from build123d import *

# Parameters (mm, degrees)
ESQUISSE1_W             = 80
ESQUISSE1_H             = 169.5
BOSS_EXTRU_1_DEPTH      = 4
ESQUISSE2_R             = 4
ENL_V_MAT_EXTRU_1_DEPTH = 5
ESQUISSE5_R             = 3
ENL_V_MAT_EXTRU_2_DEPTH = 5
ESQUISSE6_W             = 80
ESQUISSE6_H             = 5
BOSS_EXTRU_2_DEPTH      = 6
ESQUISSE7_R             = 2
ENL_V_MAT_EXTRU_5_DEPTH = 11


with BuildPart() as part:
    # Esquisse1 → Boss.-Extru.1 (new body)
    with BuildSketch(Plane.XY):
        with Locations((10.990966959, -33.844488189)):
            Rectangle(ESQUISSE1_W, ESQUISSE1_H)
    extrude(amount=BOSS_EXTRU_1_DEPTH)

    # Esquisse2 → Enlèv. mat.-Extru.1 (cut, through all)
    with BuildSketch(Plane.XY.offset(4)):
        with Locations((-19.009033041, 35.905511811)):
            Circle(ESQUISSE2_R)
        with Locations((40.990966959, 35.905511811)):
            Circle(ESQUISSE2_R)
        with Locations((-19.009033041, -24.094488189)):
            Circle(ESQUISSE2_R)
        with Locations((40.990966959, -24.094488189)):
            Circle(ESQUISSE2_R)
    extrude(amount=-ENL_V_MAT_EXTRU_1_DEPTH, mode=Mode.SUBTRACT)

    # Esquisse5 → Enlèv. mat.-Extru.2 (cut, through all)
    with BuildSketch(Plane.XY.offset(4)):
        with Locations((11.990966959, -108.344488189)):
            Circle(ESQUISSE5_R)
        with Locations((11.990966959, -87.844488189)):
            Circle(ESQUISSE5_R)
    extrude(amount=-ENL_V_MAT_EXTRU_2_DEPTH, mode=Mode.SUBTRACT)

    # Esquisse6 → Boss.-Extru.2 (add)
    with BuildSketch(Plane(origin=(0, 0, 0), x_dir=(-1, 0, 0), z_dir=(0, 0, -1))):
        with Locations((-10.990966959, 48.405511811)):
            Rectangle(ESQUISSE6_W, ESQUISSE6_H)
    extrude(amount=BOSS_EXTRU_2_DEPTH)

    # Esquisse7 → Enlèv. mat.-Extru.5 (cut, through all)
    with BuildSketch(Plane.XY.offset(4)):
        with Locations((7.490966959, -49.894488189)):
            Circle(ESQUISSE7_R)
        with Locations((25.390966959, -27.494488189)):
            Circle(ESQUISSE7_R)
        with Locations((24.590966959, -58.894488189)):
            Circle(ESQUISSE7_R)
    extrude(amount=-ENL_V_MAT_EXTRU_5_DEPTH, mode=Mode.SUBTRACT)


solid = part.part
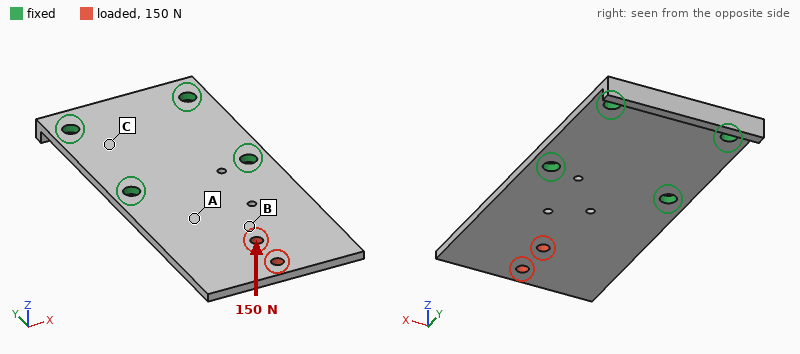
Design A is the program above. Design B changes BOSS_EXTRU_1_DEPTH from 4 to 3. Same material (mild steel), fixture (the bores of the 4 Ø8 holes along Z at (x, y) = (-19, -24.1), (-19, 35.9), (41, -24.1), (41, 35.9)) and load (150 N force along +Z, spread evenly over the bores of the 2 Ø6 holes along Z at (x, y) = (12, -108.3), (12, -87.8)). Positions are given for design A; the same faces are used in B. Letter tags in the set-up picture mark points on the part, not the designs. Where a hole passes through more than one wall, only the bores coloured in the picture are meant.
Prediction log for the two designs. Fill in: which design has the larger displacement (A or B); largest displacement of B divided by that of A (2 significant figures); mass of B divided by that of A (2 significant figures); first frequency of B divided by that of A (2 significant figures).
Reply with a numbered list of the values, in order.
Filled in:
1. B
2. 2.3
3. 0.76
4. 0.75
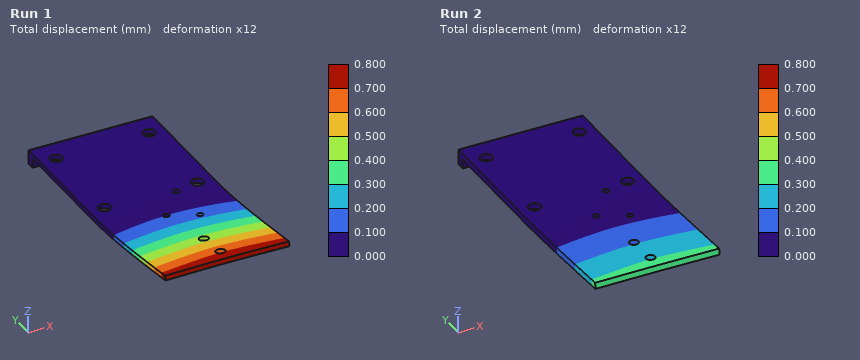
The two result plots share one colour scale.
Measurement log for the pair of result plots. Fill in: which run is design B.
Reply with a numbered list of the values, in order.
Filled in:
1. Run 1
